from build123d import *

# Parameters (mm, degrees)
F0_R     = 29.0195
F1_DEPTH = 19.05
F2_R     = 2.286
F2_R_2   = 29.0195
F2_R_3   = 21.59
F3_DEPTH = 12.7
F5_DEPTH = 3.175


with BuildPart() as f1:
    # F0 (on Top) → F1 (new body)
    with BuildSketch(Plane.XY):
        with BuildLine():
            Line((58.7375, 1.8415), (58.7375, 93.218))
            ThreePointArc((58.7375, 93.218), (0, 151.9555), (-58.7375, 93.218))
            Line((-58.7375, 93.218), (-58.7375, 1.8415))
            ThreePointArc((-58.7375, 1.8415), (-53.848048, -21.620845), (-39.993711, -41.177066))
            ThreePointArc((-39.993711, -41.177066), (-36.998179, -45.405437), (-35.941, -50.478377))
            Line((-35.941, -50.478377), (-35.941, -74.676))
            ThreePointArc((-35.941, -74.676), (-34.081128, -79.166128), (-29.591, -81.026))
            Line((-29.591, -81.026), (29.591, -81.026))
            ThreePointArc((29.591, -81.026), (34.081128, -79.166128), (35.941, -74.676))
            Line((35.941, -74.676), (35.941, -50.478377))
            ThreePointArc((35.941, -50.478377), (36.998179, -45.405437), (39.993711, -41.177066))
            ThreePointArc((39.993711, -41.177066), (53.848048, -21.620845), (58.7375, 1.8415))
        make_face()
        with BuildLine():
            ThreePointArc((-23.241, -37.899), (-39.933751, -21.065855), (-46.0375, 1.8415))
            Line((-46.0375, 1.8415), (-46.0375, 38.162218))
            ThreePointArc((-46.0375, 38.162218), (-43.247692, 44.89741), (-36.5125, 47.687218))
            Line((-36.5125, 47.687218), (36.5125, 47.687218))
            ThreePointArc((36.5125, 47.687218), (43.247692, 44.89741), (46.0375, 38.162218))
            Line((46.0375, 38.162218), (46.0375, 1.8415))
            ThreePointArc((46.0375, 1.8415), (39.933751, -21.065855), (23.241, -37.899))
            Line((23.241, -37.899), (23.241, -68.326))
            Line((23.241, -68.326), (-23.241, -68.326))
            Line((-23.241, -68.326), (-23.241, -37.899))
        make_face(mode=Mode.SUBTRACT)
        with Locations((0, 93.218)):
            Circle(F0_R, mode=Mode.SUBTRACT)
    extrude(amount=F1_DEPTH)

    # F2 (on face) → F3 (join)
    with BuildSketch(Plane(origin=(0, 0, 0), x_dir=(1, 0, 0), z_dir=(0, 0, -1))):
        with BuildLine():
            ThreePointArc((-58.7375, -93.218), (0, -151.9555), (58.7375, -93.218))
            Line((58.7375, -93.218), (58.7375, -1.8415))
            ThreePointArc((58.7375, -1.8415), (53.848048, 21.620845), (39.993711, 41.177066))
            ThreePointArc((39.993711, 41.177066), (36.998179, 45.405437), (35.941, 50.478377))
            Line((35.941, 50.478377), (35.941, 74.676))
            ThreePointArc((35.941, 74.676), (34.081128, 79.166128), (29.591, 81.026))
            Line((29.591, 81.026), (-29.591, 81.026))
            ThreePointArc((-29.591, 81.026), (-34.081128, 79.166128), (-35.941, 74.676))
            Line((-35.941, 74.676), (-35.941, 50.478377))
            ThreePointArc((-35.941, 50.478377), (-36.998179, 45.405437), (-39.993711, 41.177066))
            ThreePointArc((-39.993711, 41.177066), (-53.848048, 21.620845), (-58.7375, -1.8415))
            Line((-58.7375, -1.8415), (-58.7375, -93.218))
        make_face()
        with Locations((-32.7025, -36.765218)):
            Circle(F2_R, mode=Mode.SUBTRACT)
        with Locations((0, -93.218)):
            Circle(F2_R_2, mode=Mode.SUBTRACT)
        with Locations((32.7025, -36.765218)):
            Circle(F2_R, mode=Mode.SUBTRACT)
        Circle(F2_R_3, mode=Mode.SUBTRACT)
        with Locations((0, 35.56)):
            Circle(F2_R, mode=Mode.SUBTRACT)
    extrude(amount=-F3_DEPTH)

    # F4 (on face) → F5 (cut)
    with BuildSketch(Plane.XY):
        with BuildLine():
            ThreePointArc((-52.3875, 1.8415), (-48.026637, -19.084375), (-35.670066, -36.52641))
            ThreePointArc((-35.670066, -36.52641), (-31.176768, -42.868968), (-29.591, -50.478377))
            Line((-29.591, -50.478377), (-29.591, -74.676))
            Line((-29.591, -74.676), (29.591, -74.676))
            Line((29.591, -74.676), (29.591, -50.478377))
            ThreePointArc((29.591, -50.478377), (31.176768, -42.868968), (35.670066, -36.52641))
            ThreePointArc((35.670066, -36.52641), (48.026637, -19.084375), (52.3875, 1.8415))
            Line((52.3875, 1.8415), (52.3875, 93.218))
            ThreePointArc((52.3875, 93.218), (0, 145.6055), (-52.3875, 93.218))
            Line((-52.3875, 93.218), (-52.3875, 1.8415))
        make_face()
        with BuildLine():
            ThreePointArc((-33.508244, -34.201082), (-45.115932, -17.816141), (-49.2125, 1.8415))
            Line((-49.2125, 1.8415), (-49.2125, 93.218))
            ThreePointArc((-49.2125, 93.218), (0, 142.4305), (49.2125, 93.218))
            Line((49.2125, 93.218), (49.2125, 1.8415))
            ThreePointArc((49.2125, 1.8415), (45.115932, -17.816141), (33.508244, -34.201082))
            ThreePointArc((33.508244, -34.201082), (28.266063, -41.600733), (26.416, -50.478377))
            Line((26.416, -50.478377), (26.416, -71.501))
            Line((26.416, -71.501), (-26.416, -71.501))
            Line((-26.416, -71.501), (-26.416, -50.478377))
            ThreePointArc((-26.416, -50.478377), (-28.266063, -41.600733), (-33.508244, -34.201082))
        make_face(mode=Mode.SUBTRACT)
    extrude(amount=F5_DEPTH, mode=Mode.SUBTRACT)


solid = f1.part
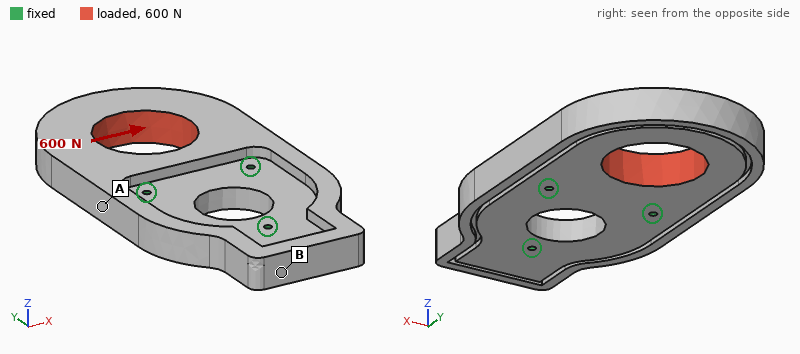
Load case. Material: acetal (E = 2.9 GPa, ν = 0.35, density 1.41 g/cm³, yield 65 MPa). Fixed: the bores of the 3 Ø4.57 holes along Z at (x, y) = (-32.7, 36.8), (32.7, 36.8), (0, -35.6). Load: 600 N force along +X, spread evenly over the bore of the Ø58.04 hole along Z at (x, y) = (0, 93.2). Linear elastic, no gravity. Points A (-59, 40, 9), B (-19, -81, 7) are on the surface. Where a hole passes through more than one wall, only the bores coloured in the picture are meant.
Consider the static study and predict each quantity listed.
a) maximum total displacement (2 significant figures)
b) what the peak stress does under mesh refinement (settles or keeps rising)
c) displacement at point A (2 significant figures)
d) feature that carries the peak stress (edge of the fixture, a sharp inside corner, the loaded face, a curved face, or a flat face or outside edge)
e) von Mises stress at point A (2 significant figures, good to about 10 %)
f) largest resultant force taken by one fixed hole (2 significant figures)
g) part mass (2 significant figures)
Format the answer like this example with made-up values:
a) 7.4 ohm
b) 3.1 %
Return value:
a) 0.10 mm
b) keeps rising
c) 0.021 mm
d) edge of the fixture
e) 1.1 MPa
f) 510 N
g) 450 g
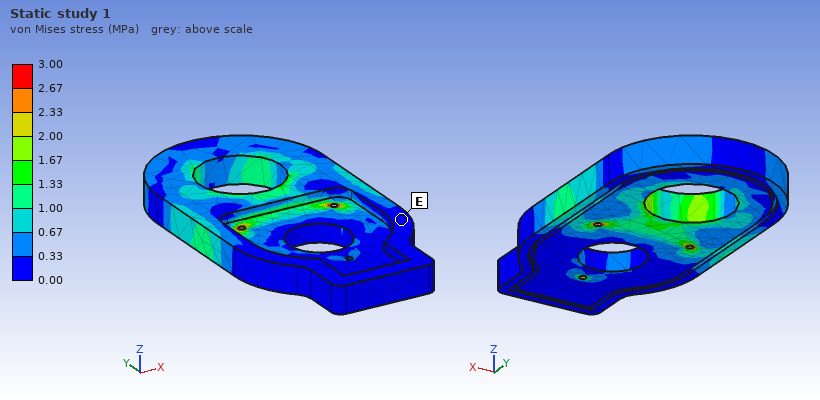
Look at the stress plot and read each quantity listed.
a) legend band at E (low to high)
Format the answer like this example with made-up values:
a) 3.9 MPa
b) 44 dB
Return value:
a) 0.00 to 0.33 MPa
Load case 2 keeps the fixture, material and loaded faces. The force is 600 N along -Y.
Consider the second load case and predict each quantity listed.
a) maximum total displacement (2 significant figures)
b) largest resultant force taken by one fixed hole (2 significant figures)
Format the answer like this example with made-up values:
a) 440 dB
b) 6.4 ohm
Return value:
a) 58 µm
b) 270 N
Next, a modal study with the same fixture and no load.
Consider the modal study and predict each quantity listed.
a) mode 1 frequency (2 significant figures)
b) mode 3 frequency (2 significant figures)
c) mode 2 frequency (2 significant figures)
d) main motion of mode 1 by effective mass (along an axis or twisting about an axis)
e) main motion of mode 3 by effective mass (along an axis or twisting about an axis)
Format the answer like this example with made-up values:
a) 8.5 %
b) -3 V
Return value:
a) 260 Hz
b) 890 Hz
c) 660 Hz
d) along Z
e) along X
